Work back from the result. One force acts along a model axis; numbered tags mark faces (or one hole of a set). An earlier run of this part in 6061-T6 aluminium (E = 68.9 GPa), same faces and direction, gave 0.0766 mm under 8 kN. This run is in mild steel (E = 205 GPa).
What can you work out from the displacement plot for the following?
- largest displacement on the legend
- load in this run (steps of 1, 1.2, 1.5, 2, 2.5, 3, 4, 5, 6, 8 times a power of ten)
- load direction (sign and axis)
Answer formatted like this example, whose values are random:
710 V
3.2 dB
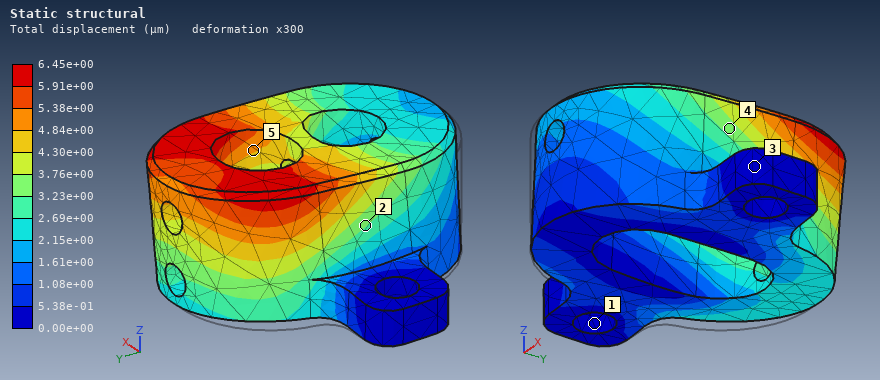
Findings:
6.45e+00 µm
2 kN
+X
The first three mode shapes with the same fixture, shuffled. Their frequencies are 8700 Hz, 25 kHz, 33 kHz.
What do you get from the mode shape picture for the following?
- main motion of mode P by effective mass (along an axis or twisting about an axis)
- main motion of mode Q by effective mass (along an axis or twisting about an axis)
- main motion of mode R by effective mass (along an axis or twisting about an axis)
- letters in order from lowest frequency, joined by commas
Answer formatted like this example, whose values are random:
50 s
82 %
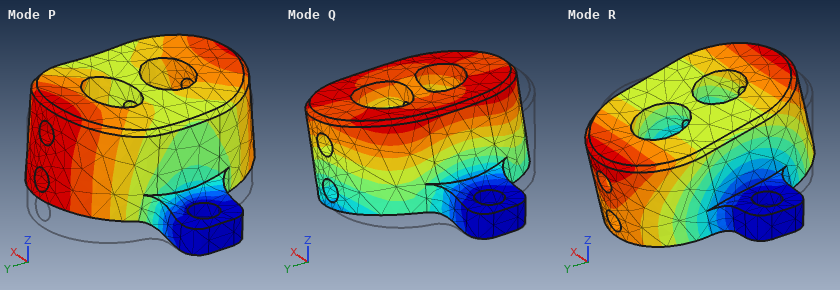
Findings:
along Z
along X
along Y
R, P, Q
